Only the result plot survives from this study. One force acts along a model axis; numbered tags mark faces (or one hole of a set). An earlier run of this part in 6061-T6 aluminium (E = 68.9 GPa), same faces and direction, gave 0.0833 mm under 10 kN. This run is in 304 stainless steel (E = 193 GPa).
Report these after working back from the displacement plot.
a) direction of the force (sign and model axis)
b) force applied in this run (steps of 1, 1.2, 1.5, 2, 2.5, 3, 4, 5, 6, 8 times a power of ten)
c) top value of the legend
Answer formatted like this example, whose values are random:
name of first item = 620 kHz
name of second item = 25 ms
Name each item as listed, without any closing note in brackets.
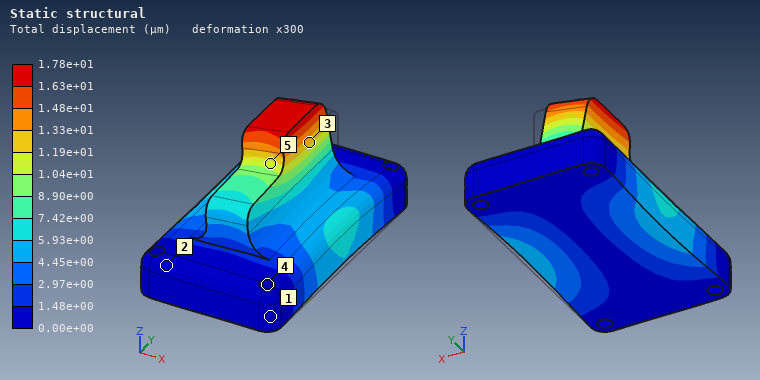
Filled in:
direction of the force = -X
force applied in this run = 6 kN
top value of the legend = 1.78e+01 µm
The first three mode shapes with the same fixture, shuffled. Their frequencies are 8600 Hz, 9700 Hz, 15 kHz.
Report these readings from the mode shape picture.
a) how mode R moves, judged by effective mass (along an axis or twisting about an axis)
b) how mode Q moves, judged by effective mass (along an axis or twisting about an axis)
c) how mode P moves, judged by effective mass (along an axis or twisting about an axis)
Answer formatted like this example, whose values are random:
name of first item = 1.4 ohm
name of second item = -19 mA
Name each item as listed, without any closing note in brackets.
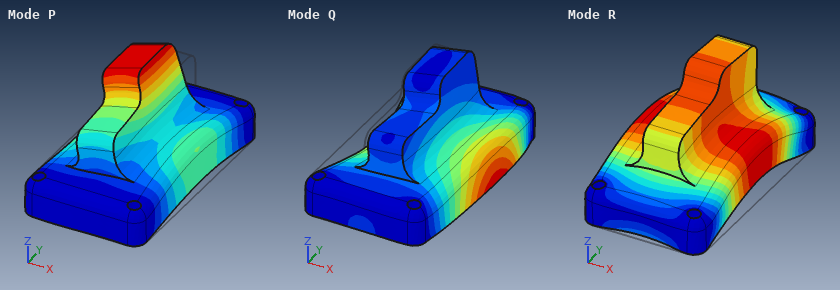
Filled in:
how mode R moves, judged by effective mass = along Z
how mode Q moves, judged by effective mass = along X
how mode P moves, judged by effective mass = along X
